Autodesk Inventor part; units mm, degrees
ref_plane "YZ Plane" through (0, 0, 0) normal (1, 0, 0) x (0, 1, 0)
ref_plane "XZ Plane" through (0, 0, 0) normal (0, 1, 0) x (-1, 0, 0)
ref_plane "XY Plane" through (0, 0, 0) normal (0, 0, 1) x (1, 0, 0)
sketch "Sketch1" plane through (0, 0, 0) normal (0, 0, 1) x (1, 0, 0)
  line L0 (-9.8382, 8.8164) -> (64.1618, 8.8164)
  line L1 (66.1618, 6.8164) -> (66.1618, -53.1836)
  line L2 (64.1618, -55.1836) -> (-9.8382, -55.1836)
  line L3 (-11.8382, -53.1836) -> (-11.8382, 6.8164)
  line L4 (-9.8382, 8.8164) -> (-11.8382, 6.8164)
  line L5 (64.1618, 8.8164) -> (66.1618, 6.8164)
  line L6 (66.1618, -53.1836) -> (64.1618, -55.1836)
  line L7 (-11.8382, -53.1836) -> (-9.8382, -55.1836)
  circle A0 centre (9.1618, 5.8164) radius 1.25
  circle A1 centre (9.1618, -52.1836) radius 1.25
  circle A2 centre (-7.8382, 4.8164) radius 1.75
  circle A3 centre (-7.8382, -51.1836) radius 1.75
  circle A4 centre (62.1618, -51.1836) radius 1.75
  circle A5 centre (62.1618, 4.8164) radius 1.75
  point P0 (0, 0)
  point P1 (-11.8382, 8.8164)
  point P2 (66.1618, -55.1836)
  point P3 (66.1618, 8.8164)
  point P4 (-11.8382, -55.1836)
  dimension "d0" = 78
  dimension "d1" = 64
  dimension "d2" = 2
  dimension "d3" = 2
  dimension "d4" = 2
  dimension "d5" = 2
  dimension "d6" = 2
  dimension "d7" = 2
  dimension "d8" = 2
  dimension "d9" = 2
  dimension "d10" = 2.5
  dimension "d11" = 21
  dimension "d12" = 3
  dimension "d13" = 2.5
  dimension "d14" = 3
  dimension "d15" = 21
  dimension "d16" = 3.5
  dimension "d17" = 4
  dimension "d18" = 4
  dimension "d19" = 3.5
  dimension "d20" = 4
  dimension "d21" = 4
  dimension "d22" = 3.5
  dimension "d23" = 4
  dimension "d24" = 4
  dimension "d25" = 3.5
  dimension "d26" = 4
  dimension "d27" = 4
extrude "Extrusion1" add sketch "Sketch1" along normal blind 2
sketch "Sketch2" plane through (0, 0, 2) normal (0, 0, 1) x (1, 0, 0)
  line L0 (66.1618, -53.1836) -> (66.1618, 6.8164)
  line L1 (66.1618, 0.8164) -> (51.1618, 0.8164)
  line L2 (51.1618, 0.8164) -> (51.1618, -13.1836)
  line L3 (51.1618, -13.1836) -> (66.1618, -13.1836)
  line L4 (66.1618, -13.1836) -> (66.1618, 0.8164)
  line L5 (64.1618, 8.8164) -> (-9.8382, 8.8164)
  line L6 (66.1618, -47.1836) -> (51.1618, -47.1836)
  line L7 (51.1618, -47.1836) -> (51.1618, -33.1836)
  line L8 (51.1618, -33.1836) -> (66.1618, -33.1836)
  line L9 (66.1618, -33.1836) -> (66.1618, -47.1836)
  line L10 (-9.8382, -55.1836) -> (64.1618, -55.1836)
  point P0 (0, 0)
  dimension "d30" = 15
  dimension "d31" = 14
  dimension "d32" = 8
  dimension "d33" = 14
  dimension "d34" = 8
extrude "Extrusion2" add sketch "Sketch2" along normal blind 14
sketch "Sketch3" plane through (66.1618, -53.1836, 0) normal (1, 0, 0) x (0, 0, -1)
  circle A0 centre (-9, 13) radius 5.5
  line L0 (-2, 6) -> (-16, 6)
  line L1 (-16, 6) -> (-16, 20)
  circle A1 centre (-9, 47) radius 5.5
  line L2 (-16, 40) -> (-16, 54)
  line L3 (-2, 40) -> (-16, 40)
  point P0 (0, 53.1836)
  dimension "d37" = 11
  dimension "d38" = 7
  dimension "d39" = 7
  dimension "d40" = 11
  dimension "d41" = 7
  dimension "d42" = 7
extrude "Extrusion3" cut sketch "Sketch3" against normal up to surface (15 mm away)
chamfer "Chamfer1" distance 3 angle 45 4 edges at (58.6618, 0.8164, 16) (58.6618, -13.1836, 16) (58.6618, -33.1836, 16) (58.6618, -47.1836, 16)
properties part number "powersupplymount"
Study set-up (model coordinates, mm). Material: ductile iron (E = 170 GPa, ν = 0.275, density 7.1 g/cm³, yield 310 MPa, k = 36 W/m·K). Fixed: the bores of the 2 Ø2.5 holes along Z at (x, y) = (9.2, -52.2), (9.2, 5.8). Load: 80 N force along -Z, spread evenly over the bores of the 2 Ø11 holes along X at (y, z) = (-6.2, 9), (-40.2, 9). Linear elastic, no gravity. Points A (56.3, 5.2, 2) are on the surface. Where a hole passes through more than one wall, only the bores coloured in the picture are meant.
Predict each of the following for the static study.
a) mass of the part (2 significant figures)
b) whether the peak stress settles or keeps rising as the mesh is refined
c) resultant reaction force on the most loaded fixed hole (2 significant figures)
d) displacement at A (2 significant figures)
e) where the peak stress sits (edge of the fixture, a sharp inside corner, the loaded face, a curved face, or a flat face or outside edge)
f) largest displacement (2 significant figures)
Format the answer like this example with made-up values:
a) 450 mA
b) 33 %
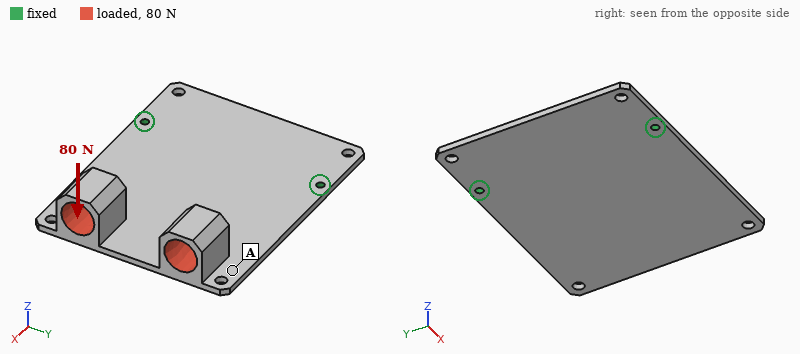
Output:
a) 90 g
b) keeps rising
c) 40 N
d) 0.60 mm
e) edge of the fixture
f) 0.83 mm
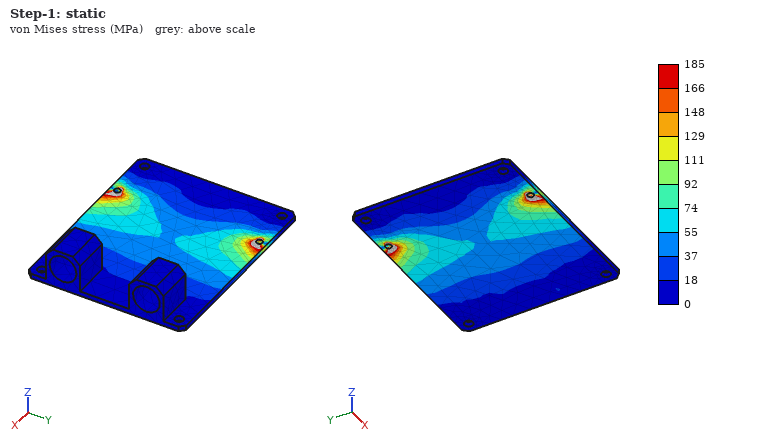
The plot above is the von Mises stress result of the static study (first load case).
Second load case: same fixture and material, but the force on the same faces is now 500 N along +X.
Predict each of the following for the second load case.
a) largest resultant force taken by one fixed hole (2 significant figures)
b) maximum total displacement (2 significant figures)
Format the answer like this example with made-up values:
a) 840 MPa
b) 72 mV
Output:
a) 250 N
b) 1.2 mm
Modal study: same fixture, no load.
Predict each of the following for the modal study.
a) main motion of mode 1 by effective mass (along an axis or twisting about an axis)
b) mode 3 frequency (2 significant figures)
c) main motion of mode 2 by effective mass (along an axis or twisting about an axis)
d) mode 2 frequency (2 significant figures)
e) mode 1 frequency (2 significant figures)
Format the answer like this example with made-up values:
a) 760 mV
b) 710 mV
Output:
a) along Z
b) 1900 Hz
c) twisting about X
d) 860 Hz
e) 280 Hz
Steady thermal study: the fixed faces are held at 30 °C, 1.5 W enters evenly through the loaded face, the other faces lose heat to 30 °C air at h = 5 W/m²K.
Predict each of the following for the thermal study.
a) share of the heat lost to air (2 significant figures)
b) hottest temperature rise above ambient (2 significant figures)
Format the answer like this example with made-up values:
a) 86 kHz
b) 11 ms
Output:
a) 33 %
b) 17 K
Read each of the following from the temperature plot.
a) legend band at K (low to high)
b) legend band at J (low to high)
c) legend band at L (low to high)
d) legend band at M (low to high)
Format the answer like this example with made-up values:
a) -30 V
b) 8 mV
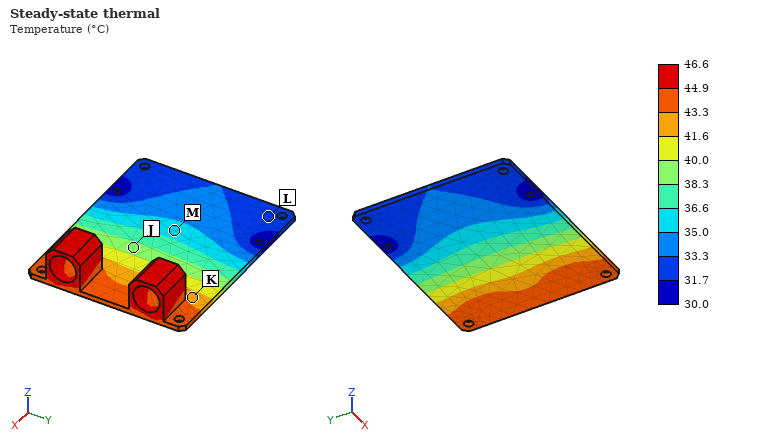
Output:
a) 41.6 to 43.3 °C
b) 38.3 to 40.0 °C
c) 31.7 to 33.3 °C
d) 35.0 to 36.6 °C
